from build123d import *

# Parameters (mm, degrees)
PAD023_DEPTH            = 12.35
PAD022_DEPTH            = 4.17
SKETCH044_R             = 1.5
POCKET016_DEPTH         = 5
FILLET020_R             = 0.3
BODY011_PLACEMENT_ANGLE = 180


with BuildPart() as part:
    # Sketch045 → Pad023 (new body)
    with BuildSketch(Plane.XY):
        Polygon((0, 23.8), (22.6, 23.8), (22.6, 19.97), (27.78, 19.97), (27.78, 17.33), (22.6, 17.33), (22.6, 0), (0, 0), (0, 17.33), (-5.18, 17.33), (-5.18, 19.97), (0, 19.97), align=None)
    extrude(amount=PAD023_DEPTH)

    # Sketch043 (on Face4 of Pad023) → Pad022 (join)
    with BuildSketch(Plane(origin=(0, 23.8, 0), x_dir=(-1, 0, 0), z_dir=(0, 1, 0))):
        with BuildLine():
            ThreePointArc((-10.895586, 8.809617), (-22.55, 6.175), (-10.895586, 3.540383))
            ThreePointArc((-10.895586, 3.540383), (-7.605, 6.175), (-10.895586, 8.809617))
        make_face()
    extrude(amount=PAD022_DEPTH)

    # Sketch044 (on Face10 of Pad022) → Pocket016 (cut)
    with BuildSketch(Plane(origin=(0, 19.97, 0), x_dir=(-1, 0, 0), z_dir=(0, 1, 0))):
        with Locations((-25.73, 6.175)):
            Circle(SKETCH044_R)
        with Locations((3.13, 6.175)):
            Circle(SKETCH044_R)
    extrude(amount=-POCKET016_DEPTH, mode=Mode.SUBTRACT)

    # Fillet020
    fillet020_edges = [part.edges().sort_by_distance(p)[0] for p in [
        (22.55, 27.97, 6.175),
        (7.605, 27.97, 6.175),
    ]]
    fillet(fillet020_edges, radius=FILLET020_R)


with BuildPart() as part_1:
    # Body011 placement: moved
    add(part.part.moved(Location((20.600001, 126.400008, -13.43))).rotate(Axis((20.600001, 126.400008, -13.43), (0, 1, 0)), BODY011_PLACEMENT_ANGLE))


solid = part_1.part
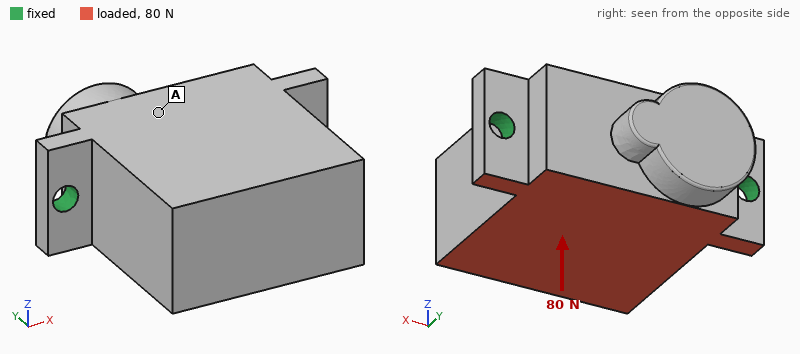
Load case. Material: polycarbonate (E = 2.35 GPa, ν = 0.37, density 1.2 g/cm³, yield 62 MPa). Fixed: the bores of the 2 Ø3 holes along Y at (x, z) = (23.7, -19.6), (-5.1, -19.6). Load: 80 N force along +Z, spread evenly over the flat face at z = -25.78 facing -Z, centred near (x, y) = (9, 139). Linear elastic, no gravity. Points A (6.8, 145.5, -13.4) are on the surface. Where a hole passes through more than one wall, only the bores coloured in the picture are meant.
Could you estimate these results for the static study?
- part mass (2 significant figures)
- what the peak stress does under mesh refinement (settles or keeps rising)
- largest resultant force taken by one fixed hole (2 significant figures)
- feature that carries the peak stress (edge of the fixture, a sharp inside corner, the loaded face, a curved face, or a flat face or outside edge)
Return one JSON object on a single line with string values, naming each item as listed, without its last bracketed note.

{"part mass": "9.0 g", "what the peak stress does under mesh refinement": "keeps rising", "largest resultant force taken by one fixed hole": "40 N", "feature that carries the peak stress": "edge of the fixture"}
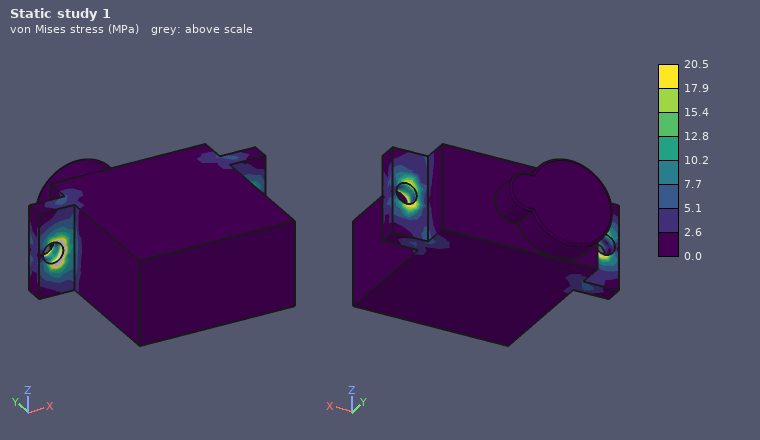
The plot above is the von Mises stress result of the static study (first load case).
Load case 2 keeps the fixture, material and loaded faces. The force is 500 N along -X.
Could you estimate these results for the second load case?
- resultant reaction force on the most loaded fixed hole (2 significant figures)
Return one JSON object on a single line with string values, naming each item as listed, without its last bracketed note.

{"resultant reaction force on the most loaded fixed hole": "300 N"}
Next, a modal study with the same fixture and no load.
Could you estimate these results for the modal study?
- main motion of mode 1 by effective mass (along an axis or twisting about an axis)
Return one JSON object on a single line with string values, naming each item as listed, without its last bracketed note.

{"main motion of mode 1 by effective mass": "along Z"}
